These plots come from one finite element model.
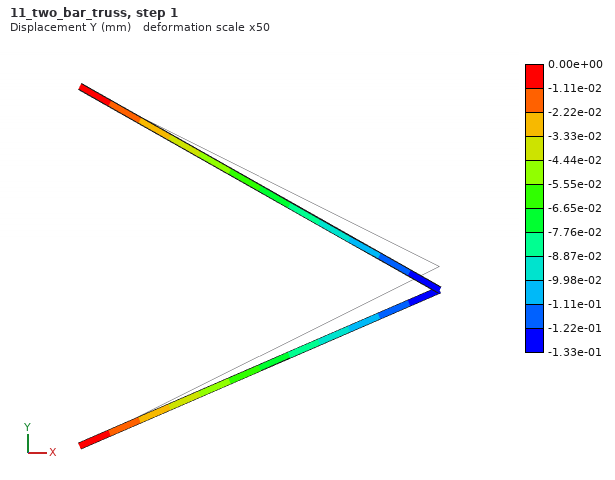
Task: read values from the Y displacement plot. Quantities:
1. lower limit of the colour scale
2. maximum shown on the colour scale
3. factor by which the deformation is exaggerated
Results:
-1.33e-01 mm
0.00e+00 mm
50
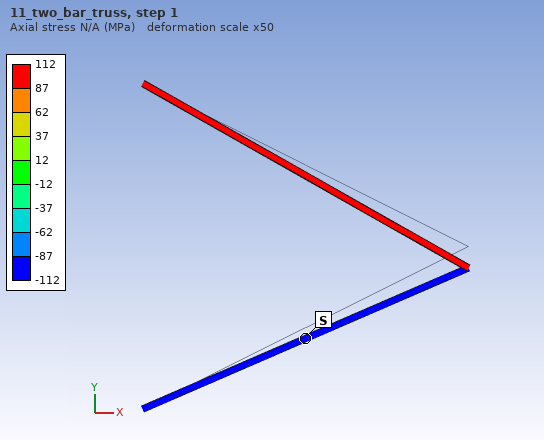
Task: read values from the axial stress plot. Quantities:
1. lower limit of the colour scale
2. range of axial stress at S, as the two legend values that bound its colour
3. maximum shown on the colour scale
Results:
-112 MPa
-112 to -87 MPa
112 MPa
